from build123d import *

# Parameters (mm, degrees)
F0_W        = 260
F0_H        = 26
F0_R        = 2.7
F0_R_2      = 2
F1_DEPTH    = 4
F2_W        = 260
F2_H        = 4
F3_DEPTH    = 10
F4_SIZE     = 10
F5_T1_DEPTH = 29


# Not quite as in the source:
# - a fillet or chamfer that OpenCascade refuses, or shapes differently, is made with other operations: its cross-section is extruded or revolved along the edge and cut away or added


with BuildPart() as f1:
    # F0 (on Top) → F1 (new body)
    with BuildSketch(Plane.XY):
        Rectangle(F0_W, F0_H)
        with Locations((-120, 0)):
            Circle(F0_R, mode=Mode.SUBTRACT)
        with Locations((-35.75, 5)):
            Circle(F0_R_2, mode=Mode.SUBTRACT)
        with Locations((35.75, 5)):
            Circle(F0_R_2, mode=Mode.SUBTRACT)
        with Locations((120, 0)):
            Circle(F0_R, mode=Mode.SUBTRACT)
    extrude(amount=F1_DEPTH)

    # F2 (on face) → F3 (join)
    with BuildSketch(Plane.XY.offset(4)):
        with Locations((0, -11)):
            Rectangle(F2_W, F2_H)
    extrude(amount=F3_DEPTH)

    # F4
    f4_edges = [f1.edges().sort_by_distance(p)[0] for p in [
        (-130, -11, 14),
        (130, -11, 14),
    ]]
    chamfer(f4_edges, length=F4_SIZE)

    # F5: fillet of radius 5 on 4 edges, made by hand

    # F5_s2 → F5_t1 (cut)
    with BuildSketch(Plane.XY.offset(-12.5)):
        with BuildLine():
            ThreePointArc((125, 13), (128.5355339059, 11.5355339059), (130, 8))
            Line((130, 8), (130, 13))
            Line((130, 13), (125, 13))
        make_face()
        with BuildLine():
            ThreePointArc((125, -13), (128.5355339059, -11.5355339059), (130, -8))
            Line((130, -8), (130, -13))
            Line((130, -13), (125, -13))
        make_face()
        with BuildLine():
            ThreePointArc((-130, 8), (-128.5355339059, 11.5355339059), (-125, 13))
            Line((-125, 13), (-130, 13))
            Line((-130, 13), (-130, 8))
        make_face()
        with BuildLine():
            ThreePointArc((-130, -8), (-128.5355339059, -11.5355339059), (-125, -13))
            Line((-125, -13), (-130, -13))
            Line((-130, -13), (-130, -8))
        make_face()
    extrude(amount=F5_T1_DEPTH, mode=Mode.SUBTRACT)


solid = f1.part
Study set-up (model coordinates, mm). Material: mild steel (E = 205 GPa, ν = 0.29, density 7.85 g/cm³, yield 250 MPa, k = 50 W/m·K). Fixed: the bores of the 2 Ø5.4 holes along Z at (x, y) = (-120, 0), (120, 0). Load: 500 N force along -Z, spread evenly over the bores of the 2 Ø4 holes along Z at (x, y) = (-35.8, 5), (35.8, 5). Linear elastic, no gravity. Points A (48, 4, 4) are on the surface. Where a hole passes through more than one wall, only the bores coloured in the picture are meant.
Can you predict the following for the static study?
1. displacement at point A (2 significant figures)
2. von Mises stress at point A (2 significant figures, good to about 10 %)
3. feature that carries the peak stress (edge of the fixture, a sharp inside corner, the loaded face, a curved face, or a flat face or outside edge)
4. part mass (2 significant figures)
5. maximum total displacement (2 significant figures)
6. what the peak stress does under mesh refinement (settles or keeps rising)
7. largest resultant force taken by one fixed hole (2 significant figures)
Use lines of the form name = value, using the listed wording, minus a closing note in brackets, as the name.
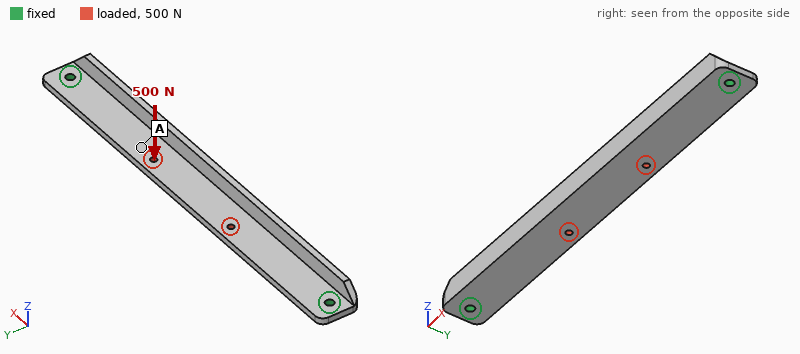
displacement at point A = 0.18 mm
von Mises stress at point A = 32 MPa
feature that carries the peak stress = edge of the fixture
part mass = 290 g
maximum total displacement = 0.27 mm
what the peak stress does under mesh refinement = keeps rising
largest resultant force taken by one fixed hole = 550 N
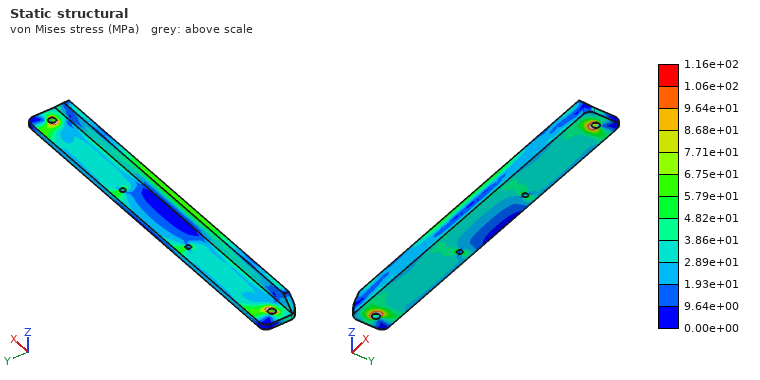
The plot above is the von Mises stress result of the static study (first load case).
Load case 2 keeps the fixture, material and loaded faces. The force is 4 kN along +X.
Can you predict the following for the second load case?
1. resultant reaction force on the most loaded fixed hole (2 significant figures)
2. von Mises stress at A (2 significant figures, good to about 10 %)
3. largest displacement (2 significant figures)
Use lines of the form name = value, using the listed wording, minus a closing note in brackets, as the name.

resultant reaction force on the most loaded fixed hole = 2.0 kN
von Mises stress at A = 24 MPa
largest displacement = 11 µm
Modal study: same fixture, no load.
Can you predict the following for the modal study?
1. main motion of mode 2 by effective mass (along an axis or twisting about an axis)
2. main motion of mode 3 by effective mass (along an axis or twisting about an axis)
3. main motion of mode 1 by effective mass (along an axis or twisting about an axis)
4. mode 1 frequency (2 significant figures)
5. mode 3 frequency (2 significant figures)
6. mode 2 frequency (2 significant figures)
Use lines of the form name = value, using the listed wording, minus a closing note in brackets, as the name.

main motion of mode 2 by effective mass = along Y
main motion of mode 3 by effective mass = twisting about Y
main motion of mode 1 by effective mass = along Z
mode 1 frequency = 680 Hz
mode 3 frequency = 1900 Hz
mode 2 frequency = 1400 Hz
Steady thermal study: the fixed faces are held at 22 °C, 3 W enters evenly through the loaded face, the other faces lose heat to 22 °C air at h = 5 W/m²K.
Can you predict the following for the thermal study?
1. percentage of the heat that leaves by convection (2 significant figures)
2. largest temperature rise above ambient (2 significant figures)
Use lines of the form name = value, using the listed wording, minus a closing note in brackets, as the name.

percentage of the heat that leaves by convection = 29 %
largest temperature rise above ambient = 16 K
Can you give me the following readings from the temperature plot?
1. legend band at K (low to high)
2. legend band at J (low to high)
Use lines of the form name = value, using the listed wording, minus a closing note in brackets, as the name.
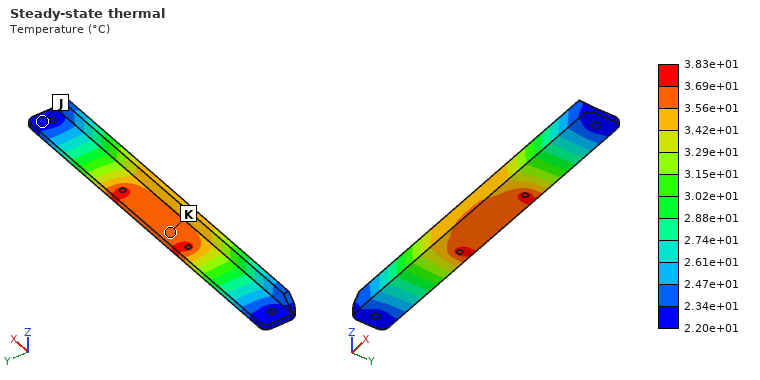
legend band at K = 3.56e+01 to 3.69e+01 °C
legend band at J = 2.20e+01 to 2.34e+01 °C
